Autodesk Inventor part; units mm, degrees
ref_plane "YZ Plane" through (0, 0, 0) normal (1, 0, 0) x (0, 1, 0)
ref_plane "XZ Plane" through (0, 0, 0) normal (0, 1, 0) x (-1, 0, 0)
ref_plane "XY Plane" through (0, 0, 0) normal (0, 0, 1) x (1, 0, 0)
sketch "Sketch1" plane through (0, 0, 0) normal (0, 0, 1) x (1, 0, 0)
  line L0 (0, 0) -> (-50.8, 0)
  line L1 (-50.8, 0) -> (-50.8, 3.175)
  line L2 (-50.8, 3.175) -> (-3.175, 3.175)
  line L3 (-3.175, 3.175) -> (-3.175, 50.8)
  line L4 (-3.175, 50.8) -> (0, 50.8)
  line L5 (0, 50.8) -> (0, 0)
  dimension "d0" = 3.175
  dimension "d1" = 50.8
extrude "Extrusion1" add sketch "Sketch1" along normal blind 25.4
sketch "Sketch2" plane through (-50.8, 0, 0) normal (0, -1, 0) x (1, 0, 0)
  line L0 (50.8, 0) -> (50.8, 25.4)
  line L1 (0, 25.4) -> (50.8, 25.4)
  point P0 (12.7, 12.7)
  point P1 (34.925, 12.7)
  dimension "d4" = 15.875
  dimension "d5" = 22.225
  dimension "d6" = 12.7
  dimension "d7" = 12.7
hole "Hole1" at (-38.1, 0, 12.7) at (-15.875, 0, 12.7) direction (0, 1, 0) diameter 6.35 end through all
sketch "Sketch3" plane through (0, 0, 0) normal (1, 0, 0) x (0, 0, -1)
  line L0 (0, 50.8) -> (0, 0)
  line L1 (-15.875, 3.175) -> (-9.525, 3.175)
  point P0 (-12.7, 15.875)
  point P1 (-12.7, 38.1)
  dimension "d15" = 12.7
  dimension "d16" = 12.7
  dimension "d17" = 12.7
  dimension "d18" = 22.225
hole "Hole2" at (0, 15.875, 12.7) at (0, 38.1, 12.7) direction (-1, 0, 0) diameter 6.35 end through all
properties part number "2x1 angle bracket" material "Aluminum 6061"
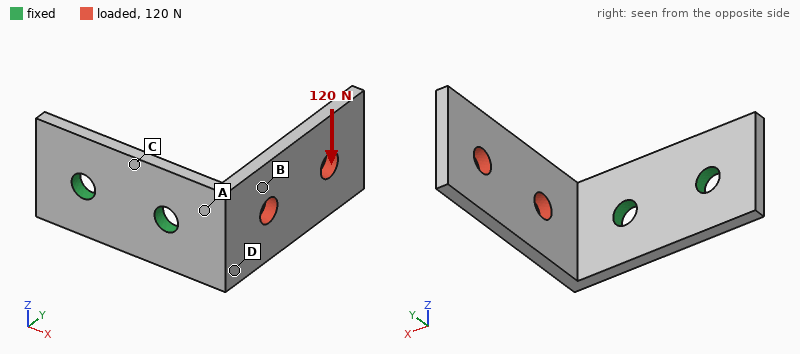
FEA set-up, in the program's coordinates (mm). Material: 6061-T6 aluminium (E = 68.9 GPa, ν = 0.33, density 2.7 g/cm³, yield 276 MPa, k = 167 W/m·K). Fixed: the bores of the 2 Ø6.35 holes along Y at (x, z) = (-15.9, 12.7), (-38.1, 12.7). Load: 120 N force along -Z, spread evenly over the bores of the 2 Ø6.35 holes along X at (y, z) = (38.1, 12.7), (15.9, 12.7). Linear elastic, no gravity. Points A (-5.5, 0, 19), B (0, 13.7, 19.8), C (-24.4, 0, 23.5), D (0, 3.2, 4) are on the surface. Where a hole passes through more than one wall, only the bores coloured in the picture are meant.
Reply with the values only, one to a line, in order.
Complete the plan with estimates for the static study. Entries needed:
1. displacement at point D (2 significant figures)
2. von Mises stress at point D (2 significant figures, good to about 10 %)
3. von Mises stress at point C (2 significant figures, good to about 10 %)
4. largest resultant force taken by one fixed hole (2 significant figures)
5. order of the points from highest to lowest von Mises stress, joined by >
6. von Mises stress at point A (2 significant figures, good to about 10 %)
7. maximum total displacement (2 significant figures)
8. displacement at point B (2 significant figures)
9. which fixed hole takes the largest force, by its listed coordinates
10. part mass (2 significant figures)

0.039 mm
25 MPa
13 MPa
160 N
A > D > C > B
31 MPa
0.22 mm
0.060 mm
(-15.9, 12.7)
20 g
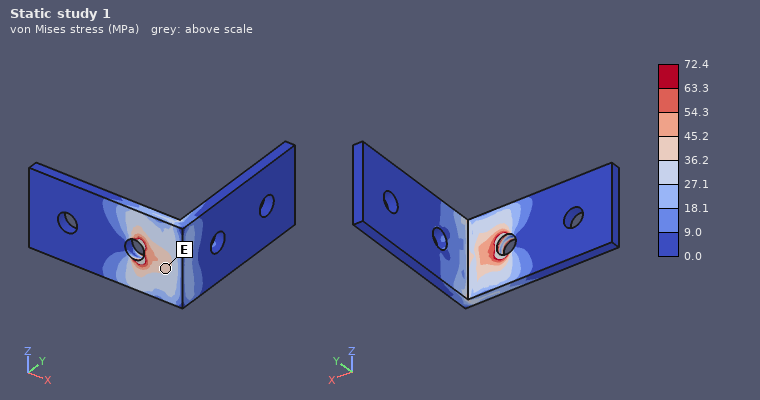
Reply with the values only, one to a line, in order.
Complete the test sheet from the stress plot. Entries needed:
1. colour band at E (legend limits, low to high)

36.2 to 45.2 MPa
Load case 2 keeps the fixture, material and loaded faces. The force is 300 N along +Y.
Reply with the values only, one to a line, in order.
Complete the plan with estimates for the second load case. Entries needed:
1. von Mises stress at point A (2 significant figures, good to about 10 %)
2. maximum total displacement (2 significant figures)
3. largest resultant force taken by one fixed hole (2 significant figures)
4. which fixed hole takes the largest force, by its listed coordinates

26 MPa
0.26 mm
330 N
(-15.9, 12.7)
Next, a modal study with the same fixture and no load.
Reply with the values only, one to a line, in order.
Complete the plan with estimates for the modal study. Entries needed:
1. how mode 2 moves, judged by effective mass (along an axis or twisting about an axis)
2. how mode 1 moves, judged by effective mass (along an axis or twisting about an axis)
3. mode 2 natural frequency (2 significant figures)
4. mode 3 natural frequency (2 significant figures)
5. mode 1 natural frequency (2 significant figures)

along Z
along X
1400 Hz
3900 Hz
770 Hz
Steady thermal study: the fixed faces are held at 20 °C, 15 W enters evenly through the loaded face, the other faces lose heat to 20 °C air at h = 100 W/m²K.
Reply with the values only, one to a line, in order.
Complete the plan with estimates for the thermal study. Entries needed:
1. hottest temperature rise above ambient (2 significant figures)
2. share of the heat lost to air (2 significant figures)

28 K
42 %
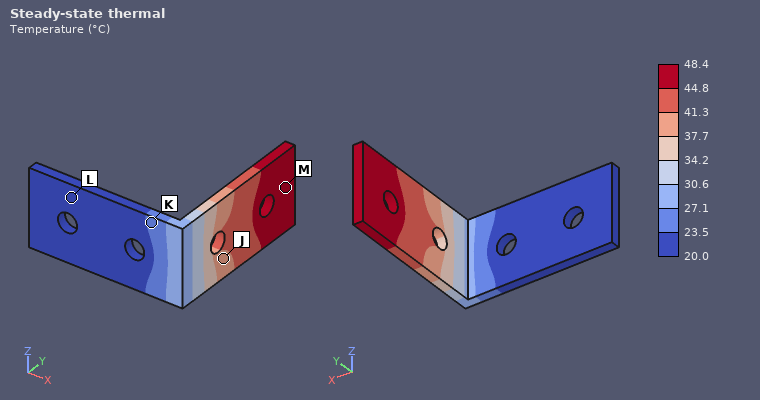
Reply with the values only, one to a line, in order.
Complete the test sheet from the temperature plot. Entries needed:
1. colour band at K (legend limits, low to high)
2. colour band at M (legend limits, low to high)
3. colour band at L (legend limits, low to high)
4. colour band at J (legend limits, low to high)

23.5 to 27.1 °C
44.8 to 48.4 °C
20.0 to 23.5 °C
37.7 to 41.3 °C
